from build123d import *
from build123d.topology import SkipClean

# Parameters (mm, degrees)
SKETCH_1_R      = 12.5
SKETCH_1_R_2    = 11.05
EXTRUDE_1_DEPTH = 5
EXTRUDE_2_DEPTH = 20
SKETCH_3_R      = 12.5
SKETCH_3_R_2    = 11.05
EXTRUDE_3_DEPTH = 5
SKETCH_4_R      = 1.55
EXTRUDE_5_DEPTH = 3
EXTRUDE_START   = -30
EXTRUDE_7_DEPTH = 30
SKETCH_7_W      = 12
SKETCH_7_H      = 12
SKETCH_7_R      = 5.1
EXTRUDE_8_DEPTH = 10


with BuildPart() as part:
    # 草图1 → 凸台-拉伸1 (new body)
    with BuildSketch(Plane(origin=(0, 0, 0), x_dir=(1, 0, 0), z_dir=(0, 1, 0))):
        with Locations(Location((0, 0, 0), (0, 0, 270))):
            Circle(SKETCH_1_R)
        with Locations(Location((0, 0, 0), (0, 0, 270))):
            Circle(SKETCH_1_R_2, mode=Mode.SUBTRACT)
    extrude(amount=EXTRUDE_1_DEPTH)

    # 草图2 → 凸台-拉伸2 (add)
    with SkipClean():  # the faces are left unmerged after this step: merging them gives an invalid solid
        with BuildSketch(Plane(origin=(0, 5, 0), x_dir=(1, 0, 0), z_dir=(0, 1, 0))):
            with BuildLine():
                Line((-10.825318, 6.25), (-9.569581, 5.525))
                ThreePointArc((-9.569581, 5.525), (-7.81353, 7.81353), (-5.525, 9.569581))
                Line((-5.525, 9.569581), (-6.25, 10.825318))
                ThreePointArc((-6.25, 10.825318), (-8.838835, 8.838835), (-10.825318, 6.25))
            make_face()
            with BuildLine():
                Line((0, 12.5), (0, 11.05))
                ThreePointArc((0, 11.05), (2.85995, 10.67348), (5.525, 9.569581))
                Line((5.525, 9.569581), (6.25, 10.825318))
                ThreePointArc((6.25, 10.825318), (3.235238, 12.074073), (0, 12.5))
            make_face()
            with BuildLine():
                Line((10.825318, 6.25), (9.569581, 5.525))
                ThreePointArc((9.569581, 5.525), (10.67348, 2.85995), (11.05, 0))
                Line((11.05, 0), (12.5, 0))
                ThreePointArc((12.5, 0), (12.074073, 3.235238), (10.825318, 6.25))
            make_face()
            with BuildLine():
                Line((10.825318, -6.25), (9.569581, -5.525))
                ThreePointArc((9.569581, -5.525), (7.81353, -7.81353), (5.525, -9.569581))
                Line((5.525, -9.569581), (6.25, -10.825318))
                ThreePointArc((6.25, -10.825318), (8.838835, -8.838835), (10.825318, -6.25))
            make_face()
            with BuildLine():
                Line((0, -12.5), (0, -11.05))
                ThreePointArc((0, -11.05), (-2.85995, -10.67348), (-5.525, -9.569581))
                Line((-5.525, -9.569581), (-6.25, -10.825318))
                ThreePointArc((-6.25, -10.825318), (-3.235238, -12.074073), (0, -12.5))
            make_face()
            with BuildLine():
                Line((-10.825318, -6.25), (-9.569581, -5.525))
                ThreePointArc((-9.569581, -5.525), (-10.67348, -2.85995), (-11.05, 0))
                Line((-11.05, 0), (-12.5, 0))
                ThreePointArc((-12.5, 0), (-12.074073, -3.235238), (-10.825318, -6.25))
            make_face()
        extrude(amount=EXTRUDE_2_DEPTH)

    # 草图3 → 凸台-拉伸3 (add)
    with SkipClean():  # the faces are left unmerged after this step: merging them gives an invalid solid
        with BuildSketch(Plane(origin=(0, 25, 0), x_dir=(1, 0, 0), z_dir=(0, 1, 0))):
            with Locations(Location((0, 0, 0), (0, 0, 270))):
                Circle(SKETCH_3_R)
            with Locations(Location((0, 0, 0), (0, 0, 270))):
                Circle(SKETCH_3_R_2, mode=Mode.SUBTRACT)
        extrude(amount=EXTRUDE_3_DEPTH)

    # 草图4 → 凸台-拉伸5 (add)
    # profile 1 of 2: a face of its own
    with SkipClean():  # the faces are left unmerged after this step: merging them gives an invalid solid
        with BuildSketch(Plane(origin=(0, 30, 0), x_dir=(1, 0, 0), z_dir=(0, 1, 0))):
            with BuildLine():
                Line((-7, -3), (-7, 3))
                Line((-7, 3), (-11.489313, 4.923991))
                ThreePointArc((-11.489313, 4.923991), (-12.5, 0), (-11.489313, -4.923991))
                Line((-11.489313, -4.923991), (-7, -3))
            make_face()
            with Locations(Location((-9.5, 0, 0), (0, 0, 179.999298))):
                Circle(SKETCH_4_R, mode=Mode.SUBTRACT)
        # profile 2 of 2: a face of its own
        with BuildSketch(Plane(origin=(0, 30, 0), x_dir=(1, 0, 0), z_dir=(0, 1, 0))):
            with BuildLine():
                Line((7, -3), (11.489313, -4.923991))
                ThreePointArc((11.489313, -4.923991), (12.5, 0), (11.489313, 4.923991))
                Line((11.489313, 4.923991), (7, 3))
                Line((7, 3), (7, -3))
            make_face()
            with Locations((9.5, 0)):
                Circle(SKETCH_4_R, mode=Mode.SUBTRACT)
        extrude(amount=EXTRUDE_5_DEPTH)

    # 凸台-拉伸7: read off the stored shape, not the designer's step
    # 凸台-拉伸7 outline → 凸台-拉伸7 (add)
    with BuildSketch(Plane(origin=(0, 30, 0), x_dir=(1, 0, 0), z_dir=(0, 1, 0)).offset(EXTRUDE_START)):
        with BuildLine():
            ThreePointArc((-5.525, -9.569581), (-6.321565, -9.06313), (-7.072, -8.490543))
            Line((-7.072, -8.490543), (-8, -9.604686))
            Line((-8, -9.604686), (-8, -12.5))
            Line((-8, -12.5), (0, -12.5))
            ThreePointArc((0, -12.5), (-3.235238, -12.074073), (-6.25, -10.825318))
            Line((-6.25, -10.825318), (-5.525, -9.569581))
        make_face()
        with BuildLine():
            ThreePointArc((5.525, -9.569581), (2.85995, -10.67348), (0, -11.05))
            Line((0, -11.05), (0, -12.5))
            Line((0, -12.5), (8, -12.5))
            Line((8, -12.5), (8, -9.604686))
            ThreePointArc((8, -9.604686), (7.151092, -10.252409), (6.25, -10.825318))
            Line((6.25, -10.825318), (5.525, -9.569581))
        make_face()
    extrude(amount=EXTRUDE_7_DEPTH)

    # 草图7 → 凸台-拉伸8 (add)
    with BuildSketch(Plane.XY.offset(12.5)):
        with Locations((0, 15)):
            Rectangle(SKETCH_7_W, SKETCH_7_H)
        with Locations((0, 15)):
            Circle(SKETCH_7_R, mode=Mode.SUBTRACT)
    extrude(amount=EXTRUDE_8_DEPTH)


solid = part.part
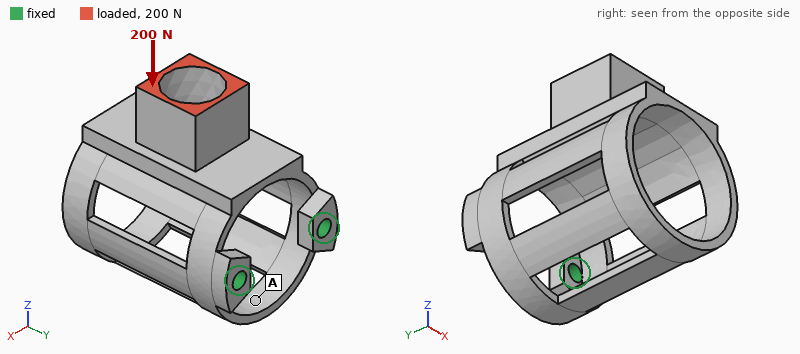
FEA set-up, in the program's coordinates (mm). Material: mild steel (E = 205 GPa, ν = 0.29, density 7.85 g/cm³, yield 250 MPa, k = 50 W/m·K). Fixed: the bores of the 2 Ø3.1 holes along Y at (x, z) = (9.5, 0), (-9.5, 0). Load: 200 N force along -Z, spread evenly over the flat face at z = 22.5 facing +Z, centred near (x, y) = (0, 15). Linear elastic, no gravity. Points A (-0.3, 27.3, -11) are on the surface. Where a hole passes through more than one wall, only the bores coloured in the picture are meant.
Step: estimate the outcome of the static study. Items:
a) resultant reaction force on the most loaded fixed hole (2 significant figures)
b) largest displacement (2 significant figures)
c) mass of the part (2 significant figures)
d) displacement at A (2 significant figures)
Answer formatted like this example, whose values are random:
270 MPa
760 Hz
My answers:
110 N
43 µm
29 g
9.4 µm
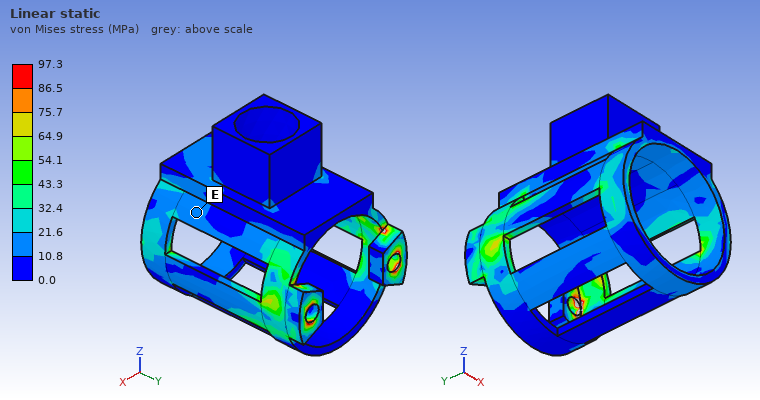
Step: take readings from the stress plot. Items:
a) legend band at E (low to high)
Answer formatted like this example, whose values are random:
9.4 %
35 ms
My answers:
10.8 to 21.6 MPa
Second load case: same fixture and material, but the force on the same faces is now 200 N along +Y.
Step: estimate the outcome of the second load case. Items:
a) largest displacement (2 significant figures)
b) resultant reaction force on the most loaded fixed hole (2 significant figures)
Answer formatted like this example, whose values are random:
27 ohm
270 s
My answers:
59 µm
110 N
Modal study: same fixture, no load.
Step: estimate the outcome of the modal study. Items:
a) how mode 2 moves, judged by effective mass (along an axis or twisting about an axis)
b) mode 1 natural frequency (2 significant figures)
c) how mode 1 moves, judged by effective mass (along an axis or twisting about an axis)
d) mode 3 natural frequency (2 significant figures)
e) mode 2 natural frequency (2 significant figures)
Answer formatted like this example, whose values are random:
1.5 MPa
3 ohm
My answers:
along X
2400 Hz
along Z
5900 Hz
5000 Hz
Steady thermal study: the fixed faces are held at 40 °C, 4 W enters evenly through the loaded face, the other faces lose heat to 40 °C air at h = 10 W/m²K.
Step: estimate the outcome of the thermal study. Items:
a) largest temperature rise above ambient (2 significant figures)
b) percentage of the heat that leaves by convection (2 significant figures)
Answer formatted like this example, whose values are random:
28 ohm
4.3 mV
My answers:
49 K
29 %
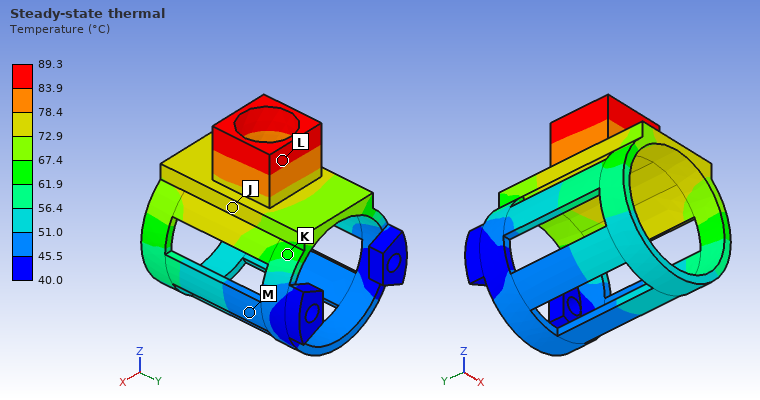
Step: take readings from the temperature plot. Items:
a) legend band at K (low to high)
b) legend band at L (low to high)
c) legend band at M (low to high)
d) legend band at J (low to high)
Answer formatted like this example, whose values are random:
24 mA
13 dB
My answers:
61.9 to 67.4 °C
83.9 to 89.3 °C
45.5 to 51.0 °C
72.9 to 78.4 °C
